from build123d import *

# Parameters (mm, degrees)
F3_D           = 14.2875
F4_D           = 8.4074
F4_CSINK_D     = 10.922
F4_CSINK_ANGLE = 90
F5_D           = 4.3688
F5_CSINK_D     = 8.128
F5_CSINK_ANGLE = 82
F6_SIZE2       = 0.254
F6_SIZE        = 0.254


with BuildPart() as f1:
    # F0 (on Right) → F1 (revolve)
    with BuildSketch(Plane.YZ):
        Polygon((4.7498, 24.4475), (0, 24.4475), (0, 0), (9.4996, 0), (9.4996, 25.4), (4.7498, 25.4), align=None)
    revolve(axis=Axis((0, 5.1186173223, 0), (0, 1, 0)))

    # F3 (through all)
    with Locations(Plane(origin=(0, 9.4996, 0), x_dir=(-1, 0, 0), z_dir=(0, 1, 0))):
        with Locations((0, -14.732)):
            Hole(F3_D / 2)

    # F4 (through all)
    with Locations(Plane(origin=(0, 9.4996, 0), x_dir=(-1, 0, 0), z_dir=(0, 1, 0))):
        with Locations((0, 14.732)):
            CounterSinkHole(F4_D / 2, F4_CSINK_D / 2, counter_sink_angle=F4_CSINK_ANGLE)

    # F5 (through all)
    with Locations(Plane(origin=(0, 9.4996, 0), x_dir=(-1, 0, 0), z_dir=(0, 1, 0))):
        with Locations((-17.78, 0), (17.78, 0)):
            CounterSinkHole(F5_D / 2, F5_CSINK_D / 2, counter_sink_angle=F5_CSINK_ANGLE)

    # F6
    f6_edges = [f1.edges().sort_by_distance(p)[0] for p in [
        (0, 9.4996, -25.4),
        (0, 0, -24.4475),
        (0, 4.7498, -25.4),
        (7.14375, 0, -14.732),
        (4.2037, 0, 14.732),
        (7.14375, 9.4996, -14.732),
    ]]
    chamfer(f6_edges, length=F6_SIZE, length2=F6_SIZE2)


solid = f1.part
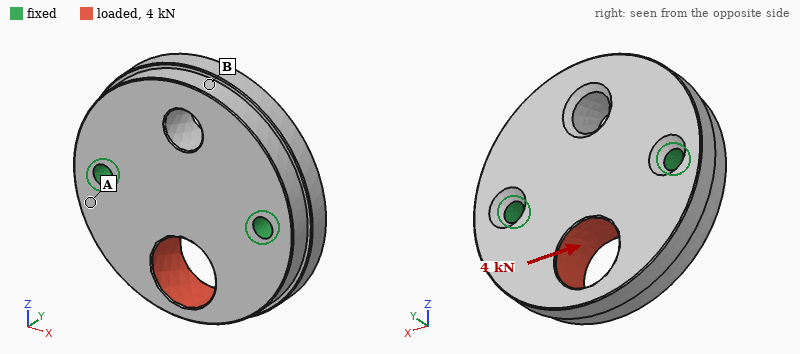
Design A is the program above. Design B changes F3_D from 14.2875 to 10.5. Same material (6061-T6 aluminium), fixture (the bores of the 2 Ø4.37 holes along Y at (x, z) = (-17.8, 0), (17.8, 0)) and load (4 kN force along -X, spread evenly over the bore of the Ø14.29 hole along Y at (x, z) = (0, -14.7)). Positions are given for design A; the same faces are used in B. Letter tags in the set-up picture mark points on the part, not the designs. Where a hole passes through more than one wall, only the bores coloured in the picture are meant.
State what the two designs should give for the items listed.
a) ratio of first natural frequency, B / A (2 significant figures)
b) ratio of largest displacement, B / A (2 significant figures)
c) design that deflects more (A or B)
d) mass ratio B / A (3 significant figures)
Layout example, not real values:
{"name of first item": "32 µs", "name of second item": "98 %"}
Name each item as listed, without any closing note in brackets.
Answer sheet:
{"ratio of first natural frequency, B / A": "0.97", "ratio of largest displacement, B / A": "0.72", "design that deflects more": "A", "mass ratio B / A": "1.04"}
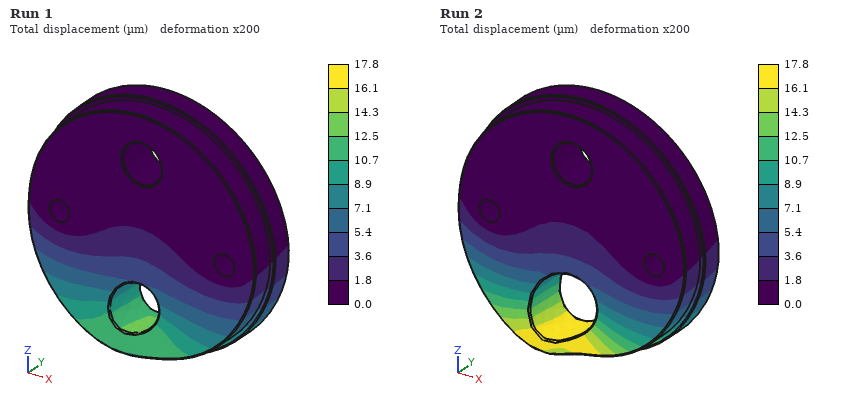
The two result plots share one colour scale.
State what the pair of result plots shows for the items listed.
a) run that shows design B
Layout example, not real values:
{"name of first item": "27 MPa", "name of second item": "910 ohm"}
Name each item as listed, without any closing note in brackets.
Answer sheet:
{"run that shows design B": "Run 1"}
